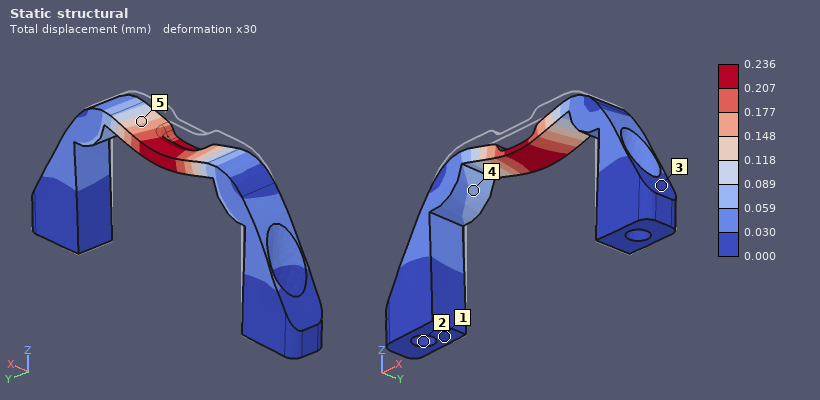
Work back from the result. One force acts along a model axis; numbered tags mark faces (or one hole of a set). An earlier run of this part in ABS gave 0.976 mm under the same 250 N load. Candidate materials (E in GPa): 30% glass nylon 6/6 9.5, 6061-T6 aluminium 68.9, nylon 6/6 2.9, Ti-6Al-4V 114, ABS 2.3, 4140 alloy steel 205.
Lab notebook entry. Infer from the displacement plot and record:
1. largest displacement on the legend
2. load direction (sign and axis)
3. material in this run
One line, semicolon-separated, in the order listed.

0.236 mm; -Z; 30% glass nylon 6/6
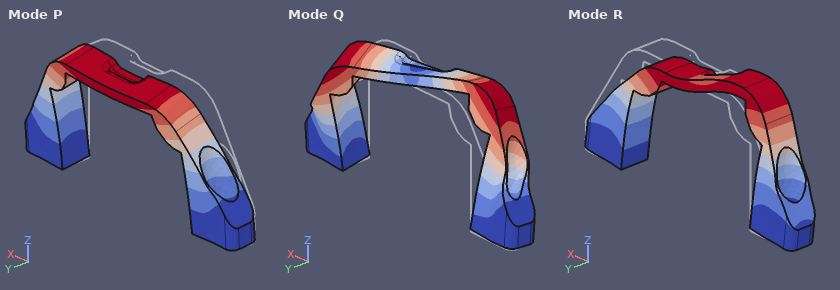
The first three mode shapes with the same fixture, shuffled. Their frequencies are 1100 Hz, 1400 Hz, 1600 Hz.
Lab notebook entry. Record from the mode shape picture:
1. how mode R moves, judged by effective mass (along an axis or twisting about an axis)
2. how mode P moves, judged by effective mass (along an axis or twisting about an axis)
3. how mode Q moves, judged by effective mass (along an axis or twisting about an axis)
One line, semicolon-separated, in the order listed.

along X; along Y; twisting about Z
